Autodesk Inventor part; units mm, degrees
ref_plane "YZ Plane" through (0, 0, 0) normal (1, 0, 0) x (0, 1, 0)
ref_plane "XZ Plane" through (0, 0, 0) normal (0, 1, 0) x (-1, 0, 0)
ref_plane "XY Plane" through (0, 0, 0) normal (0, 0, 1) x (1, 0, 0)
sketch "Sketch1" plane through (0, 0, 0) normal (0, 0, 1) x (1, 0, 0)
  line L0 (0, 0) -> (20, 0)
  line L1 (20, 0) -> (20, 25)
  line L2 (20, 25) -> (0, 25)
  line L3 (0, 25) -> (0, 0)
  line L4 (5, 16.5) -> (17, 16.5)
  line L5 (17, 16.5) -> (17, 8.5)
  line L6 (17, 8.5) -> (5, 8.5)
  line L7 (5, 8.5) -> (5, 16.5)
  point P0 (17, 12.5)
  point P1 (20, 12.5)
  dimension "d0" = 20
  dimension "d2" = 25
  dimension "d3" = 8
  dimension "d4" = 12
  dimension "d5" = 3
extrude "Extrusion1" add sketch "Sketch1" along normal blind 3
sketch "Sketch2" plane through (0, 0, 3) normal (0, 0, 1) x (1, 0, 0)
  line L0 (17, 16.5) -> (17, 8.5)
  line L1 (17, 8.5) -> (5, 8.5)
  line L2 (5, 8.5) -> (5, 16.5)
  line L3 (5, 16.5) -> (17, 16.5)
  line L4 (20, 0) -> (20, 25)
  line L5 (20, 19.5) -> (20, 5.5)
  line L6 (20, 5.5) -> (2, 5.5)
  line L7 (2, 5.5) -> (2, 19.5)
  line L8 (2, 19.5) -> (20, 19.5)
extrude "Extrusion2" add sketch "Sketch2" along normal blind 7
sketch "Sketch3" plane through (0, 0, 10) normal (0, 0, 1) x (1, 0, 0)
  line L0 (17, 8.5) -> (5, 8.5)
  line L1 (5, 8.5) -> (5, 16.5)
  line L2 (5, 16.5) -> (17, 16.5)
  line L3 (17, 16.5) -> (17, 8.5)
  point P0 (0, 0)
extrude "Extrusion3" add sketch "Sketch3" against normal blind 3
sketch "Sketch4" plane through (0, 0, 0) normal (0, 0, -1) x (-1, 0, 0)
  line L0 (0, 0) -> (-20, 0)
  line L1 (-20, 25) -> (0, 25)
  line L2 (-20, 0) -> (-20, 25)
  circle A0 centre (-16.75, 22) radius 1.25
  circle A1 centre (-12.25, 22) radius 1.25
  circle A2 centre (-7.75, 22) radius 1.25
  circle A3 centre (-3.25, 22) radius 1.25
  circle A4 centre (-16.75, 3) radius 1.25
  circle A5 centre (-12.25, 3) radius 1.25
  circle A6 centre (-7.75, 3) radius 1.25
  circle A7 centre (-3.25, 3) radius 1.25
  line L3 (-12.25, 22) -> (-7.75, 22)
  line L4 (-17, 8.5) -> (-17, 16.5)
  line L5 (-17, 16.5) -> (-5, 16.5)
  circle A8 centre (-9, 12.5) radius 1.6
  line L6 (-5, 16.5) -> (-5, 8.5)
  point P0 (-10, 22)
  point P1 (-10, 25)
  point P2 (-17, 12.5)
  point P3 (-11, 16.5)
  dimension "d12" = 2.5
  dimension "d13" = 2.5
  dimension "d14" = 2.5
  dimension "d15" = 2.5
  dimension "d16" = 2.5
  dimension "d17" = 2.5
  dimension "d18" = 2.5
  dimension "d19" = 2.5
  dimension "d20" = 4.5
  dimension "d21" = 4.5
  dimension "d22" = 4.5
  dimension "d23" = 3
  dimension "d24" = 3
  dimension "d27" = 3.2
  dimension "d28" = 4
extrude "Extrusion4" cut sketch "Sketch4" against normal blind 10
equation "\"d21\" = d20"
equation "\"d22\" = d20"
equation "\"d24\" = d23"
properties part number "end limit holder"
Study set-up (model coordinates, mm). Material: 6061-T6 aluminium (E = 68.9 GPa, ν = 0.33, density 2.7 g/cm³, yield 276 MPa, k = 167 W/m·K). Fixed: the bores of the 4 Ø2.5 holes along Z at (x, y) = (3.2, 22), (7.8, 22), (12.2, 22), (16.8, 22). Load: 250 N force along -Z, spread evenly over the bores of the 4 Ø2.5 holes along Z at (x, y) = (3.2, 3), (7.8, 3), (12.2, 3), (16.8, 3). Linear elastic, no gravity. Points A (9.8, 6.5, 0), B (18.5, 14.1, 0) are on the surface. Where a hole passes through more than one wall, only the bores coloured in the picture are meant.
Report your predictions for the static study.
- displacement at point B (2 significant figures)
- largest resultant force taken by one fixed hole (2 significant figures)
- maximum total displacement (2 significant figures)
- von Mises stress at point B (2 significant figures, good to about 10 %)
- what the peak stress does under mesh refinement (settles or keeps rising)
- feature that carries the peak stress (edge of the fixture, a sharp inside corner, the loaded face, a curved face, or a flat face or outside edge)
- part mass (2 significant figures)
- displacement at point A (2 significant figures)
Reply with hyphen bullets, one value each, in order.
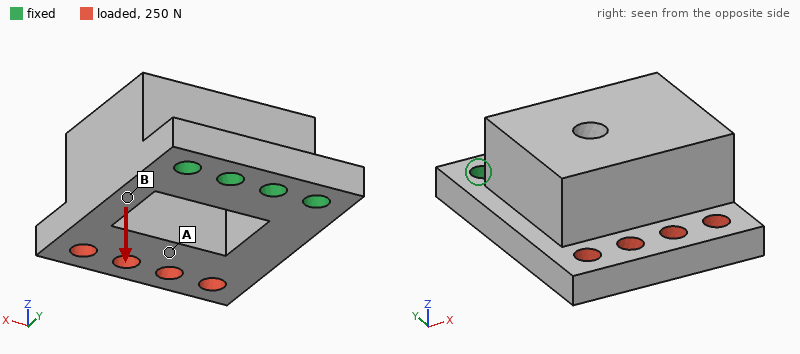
- 0.031 mm
- 130 N
- 0.12 mm
- 32 MPa
- keeps rising
- edge of the fixture
- 6.6 g
- 0.074 mm
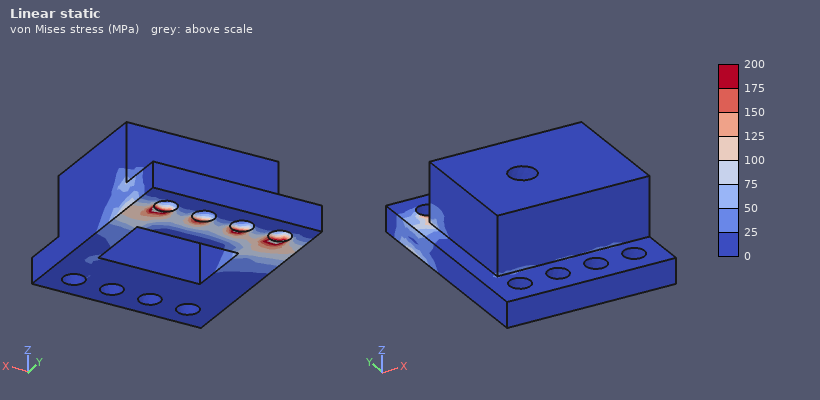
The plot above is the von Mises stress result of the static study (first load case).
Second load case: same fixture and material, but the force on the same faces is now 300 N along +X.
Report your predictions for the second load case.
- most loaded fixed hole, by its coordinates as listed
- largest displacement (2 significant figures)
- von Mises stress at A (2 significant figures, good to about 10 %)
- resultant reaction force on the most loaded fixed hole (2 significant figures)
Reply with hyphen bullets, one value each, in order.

- (3.2, 22)
- 32 µm
- 19 MPa
- 380 N
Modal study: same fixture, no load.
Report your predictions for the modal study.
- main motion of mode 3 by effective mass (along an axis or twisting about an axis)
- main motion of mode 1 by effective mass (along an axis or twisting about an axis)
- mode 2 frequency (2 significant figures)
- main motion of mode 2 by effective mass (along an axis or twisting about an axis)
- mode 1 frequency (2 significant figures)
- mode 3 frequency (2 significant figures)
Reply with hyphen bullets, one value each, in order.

- along X
- along Z
- 12 kHz
- along X
- 5300 Hz
- 20 kHz
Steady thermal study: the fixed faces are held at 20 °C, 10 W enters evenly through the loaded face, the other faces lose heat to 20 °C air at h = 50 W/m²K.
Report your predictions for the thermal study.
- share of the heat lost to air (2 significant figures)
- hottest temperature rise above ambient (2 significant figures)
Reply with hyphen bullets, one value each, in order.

- 7.5 %
- 18 K
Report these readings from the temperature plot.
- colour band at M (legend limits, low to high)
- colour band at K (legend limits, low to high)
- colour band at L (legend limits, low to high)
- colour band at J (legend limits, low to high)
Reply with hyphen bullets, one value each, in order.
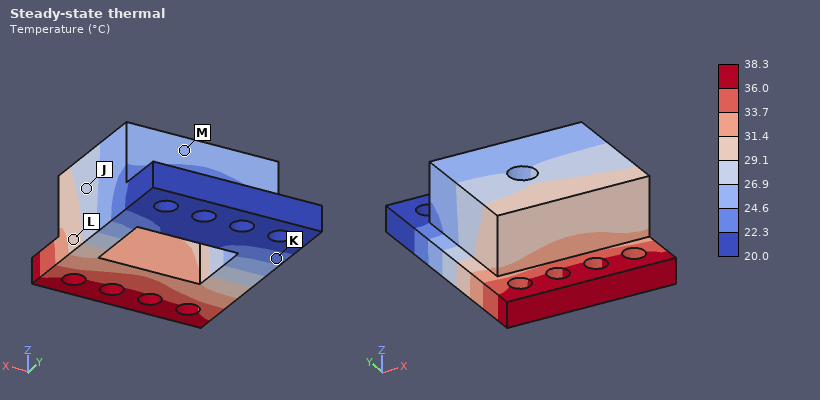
- 24.6 to 26.9 °C
- 22.3 to 24.6 °C
- 29.1 to 31.4 °C
- 26.9 to 29.1 °C
